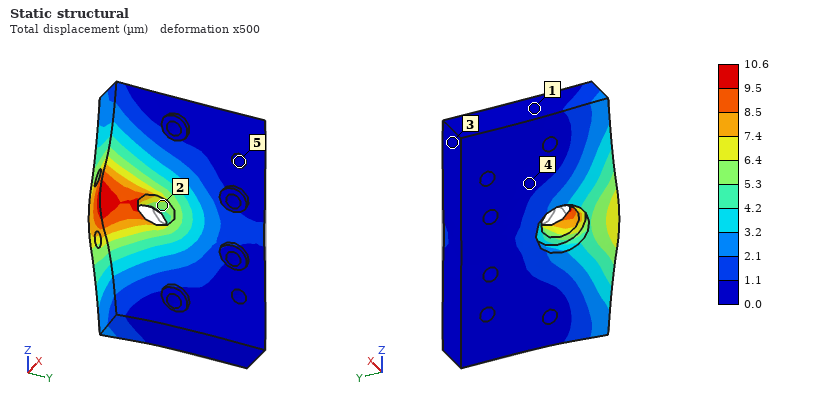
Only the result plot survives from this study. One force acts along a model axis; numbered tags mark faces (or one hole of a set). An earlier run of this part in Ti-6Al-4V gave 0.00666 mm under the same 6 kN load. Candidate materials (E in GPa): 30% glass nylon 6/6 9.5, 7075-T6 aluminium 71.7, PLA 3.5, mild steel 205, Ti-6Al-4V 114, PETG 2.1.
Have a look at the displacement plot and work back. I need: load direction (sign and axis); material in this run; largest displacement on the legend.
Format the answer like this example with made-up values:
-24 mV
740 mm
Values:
-Y
7075-T6 aluminium
10.6 µm
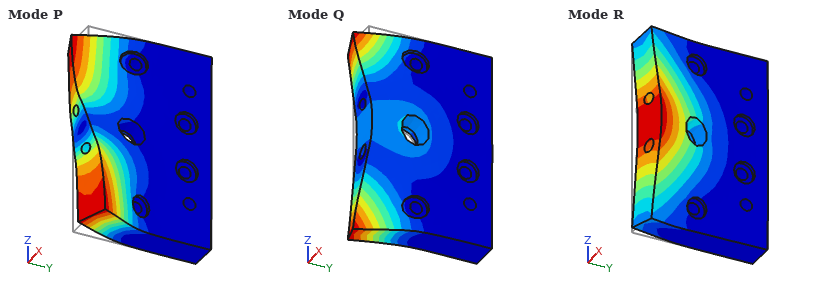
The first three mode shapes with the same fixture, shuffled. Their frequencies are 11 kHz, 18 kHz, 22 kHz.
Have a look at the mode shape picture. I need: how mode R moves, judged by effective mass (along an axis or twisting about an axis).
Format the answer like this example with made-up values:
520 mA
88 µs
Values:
along X
